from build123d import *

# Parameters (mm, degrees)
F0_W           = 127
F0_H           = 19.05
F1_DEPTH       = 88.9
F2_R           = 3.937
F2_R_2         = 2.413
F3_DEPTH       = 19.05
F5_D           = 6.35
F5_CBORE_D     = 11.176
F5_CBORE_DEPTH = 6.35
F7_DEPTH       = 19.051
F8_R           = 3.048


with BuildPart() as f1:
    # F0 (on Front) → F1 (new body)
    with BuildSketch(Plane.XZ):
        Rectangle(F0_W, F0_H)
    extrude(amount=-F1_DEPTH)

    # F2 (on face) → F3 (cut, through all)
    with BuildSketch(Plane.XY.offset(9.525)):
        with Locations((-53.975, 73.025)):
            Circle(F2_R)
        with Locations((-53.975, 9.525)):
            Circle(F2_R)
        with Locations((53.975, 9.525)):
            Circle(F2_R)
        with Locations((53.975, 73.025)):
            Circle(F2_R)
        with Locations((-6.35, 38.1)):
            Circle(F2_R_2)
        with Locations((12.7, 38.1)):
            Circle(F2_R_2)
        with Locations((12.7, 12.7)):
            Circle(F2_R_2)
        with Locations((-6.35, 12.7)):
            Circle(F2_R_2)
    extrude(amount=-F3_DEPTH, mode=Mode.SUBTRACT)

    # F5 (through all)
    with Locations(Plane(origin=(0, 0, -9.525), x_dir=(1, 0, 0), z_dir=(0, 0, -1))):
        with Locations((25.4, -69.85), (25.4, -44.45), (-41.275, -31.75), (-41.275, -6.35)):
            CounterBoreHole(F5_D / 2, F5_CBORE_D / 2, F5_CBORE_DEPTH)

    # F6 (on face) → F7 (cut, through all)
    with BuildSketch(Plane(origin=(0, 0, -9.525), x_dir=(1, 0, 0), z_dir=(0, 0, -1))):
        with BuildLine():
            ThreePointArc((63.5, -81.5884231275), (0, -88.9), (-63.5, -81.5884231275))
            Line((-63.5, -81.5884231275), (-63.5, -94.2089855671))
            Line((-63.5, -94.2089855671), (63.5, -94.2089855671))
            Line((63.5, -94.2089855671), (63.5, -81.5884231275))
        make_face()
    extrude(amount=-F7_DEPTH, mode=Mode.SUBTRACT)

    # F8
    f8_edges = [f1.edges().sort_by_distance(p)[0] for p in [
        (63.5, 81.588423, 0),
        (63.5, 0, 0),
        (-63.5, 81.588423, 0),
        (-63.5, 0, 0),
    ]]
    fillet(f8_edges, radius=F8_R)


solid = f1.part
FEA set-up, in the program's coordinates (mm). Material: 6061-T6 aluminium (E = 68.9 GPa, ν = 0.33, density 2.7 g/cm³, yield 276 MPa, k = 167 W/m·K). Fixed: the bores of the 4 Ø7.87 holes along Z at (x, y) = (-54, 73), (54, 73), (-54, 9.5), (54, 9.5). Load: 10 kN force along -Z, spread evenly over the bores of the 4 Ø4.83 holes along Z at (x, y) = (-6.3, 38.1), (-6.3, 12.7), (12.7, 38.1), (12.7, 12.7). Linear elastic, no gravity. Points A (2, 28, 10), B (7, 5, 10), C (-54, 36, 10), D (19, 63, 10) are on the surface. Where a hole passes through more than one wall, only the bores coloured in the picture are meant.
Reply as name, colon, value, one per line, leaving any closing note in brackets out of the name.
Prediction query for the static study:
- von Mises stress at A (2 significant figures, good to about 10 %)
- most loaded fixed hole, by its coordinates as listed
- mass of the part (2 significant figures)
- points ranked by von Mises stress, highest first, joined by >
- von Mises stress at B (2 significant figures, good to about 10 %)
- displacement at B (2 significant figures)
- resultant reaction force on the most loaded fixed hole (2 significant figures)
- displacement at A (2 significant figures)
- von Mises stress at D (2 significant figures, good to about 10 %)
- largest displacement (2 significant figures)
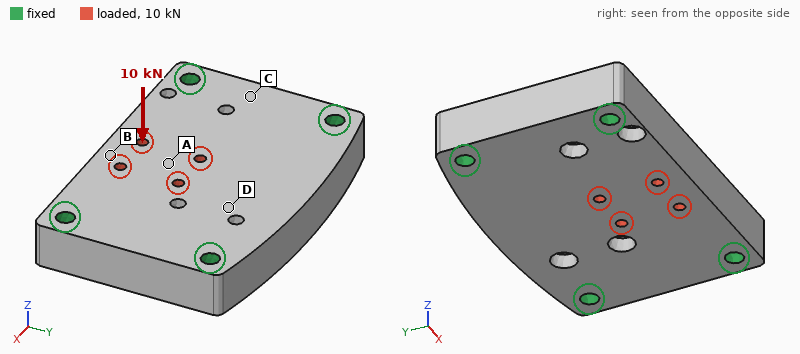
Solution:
von Mises stress at A: 26 MPa
most loaded fixed hole, by its coordinates as listed: (54, 9.5)
mass of the part: 540 g
points ranked by von Mises stress, highest first, joined by >: B > A > D > C
von Mises stress at B: 33 MPa
displacement at B: 46 µm
resultant reaction force on the most loaded fixed hole: 4.1 kN
displacement at A: 40 µm
von Mises stress at D: 12 MPa
largest displacement: 51 µm
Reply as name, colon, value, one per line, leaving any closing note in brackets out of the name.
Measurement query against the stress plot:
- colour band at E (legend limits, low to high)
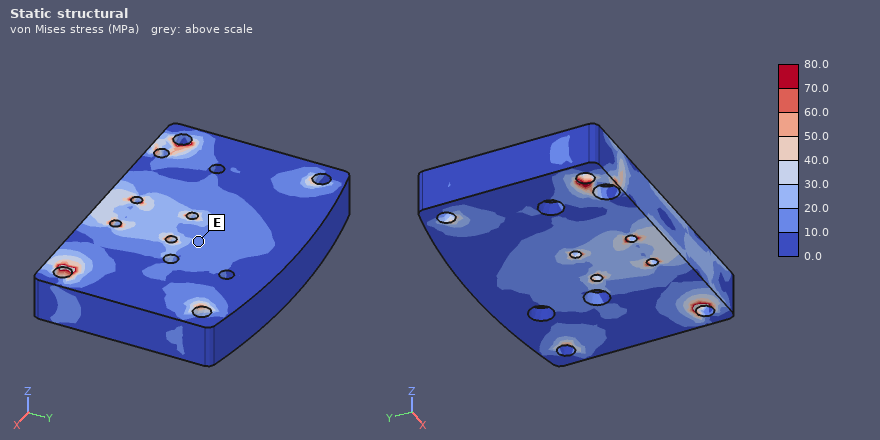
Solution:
colour band at E: 10.0 to 20.0 MPa
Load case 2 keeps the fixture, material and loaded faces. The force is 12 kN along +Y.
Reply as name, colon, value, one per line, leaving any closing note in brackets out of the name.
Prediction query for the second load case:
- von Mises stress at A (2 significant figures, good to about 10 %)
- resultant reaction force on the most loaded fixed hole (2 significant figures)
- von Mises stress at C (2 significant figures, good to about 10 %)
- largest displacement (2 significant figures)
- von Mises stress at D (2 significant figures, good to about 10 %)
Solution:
von Mises stress at A: 5.3 MPa
resultant reaction force on the most loaded fixed hole: 4.0 kN
von Mises stress at C: 2.9 MPa
largest displacement: 12 µm
von Mises stress at D: 5.1 MPa
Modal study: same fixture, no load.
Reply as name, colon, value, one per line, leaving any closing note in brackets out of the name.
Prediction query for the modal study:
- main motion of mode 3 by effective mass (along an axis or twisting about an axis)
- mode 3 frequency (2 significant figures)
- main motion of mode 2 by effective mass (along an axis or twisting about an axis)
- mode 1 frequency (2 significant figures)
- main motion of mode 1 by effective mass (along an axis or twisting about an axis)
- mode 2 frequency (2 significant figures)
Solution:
main motion of mode 3 by effective mass: along Y
mode 3 frequency: 12 kHz
main motion of mode 2 by effective mass: twisting about X
mode 1 frequency: 6000 Hz
main motion of mode 1 by effective mass: along Z
mode 2 frequency: 8200 Hz
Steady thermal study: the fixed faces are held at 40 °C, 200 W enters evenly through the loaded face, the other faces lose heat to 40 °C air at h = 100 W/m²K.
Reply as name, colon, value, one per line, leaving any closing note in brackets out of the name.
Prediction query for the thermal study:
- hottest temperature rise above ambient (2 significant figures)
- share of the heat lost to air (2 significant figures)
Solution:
hottest temperature rise above ambient: 27 K
share of the heat lost to air: 14 %
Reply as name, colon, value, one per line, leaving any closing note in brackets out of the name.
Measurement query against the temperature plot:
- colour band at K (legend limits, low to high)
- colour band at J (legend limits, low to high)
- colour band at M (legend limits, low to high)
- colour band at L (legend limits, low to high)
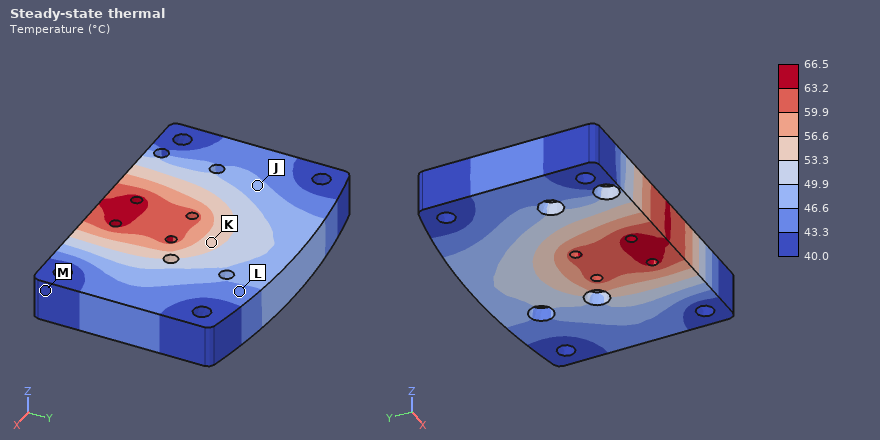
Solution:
colour band at K: 53.3 to 56.6 °C
colour band at J: 46.6 to 49.9 °C
colour band at M: 40.0 to 43.3 °C
colour band at L: 43.3 to 46.6 °C
